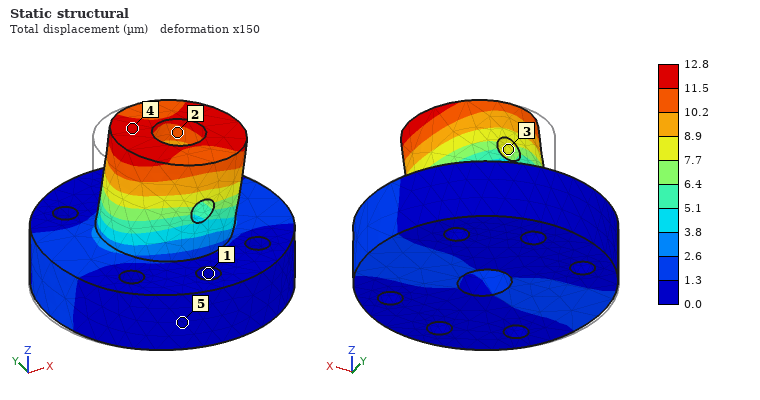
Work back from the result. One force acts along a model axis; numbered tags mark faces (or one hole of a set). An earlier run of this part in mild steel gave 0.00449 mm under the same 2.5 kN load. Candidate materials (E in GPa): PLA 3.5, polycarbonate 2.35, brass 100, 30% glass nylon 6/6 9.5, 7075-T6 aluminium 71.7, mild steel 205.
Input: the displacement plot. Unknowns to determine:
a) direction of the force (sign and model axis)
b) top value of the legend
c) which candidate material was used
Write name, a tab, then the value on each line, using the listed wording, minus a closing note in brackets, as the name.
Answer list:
direction of the force	+X
top value of the legend	12.8 µm
which candidate material was used	7075-T6 aluminium
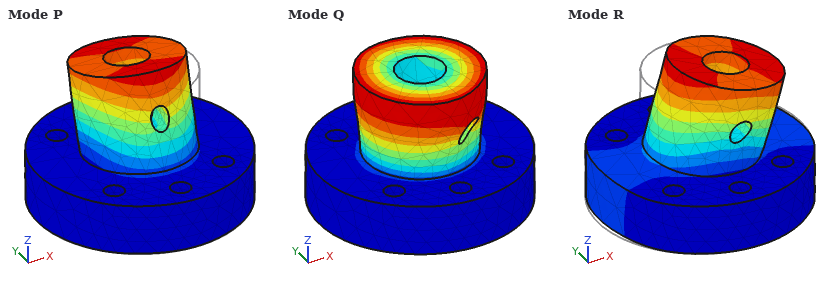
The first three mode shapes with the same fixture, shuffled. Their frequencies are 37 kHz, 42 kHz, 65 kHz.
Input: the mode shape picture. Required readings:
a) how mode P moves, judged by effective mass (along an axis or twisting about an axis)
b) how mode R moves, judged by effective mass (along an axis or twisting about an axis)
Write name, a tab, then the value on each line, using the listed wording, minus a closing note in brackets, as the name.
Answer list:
how mode P moves, judged by effective mass	along Y
how mode R moves, judged by effective mass	along X
